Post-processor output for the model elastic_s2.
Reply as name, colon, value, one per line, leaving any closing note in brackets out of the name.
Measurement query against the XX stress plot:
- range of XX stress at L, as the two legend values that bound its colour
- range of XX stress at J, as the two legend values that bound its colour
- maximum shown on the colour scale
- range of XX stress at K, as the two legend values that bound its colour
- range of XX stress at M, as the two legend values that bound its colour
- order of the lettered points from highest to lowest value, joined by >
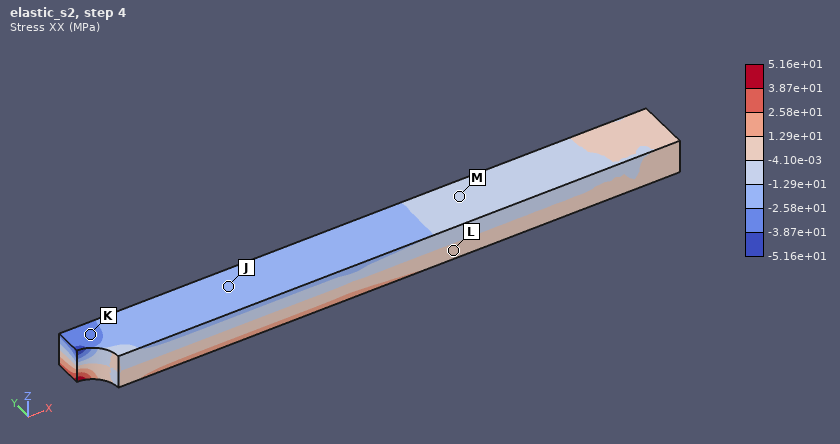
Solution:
range of XX stress at L, as the two legend values that bound its colour: -4.10e-03 to 1.29e+01 MPa
range of XX stress at J, as the two legend values that bound its colour: -2.58e+01 to -1.29e+01 MPa
maximum shown on the colour scale: 5.16e+01 MPa
range of XX stress at K, as the two legend values that bound its colour: -3.87e+01 to -2.58e+01 MPa
range of XX stress at M, as the two legend values that bound its colour: -1.29e+01 to -4.10e-03 MPa
order of the lettered points from highest to lowest value, joined by >: L > M > J > K
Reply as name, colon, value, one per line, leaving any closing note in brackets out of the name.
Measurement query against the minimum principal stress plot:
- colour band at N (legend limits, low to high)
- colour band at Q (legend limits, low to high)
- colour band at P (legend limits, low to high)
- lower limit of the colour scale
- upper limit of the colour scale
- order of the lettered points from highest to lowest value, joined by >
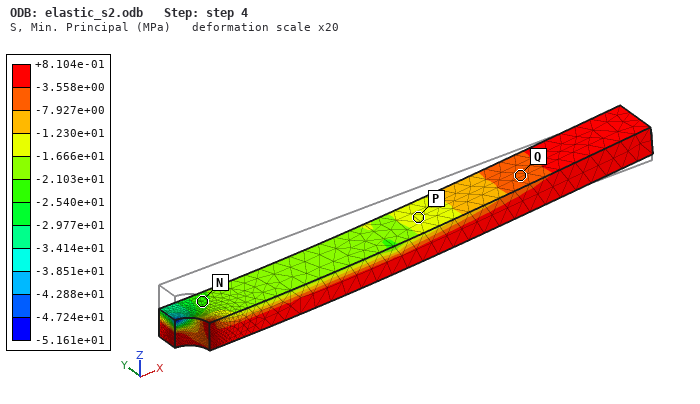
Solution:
colour band at N: -2.540e+01 to -2.103e+01 MPa
colour band at Q: -7.927e+00 to -3.558e+00 MPa
colour band at P: -1.666e+01 to -1.230e+01 MPa
lower limit of the colour scale: -5.161e+01 MPa
upper limit of the colour scale: +8.104e-01 MPa
order of the lettered points from highest to lowest value, joined by >: Q > P > N
